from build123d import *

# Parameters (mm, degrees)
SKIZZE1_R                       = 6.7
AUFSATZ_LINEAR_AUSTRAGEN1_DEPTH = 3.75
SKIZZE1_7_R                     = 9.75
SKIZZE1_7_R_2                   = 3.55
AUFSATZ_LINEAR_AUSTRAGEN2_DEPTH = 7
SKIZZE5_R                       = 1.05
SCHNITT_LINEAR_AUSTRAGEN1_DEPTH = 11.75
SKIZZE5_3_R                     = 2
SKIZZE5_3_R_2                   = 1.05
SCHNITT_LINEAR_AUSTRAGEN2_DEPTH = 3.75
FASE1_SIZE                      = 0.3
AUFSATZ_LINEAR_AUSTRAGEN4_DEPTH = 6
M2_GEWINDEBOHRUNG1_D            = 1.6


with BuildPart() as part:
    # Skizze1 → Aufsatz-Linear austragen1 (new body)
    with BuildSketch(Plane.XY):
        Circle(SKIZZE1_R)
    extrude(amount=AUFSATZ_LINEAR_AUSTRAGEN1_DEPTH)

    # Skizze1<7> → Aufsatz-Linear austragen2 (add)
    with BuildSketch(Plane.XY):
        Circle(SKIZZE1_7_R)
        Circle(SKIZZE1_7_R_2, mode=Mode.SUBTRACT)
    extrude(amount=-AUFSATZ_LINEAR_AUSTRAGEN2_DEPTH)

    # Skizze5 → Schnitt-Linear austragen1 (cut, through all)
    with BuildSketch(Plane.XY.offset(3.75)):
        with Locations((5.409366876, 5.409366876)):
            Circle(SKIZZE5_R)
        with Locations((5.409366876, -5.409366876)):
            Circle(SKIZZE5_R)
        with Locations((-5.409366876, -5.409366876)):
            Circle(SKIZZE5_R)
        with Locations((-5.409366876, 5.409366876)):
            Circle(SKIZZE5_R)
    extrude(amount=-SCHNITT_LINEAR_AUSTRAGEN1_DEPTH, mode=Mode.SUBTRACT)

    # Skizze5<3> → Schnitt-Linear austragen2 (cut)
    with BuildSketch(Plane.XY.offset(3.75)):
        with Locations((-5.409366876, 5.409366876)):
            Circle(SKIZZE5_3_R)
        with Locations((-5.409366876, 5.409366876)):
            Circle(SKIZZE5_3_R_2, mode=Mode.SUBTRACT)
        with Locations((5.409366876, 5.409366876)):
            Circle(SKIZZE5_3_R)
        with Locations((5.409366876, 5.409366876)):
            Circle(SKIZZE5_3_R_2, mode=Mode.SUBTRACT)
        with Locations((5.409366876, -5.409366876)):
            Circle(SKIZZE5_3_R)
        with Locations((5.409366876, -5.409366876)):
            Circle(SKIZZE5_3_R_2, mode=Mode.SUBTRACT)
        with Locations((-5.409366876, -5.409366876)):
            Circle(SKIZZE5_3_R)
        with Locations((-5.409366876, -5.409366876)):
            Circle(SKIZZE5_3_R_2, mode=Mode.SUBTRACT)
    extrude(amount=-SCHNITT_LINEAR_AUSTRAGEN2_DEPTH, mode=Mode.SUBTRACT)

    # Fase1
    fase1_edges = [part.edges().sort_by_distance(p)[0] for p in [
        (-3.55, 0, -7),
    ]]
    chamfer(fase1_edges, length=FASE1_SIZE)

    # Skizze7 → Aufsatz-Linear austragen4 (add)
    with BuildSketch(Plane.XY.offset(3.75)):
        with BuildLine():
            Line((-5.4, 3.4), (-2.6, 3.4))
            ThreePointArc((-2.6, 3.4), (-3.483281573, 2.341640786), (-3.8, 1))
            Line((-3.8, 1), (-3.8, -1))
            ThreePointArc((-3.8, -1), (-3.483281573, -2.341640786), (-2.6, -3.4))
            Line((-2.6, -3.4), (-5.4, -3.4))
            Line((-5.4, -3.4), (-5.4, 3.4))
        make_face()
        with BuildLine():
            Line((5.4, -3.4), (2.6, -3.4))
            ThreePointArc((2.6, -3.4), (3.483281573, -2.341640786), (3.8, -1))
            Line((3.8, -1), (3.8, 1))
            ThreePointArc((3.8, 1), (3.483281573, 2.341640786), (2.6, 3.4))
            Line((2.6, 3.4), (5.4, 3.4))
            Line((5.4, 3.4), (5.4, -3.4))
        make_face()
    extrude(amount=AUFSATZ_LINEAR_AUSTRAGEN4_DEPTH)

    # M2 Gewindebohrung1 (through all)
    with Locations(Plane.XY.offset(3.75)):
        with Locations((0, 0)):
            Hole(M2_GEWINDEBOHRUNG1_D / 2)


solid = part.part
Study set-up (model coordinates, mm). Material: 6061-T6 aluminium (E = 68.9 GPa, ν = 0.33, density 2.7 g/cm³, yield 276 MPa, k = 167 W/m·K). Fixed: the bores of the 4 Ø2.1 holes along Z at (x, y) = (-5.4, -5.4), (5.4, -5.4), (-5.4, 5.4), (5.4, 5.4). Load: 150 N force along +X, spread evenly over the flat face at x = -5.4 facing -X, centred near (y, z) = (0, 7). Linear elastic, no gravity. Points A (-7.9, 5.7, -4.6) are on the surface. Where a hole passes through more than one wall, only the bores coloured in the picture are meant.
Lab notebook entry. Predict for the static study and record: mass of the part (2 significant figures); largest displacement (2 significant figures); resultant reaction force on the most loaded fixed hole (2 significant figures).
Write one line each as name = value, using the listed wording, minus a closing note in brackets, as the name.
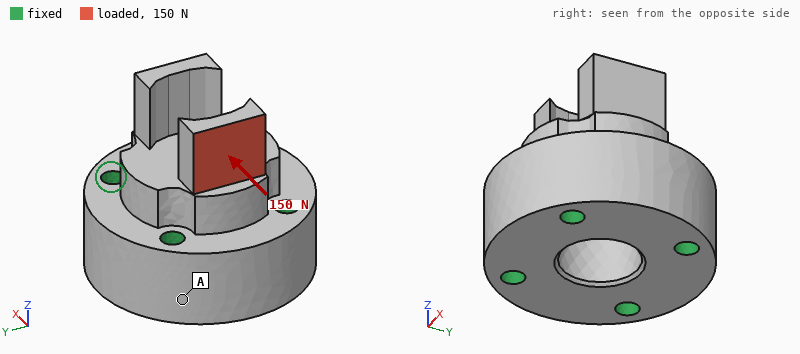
mass of the part = 6.4 g
largest displacement = 24 µm
resultant reaction force on the most loaded fixed hole = 77 N
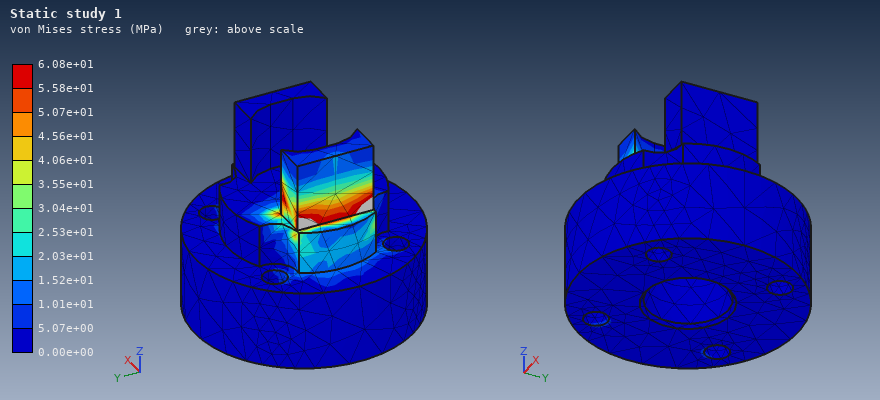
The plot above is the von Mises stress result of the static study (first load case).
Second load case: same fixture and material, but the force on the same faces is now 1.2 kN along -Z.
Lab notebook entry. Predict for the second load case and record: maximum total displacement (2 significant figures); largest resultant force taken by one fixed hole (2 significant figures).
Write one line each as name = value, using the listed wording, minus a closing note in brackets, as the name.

maximum total displacement = 72 µm
largest resultant force taken by one fixed hole = 610 N
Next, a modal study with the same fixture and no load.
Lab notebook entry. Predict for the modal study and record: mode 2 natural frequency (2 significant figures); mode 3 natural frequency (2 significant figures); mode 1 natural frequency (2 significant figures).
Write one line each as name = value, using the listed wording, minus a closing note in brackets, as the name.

mode 2 natural frequency = 35 kHz
mode 3 natural frequency = 54 kHz
mode 1 natural frequency = 34 kHz
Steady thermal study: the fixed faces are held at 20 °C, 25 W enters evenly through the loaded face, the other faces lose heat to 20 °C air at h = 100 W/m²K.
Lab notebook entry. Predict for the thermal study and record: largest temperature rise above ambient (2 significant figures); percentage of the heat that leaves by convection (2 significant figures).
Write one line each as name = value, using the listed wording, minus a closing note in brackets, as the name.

largest temperature rise above ambient = 60 K
percentage of the heat that leaves by convection = 3.1 %
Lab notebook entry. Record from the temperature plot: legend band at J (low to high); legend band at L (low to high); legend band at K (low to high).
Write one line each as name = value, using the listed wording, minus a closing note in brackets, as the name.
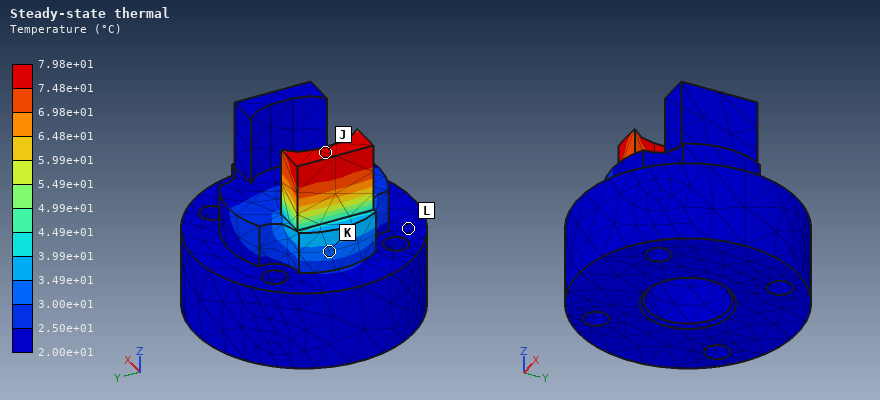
legend band at J = 7.48e+01 to 7.98e+01 °C
legend band at L = 2.00e+01 to 2.50e+01 °C
legend band at K = 3.00e+01 to 3.49e+01 °C
